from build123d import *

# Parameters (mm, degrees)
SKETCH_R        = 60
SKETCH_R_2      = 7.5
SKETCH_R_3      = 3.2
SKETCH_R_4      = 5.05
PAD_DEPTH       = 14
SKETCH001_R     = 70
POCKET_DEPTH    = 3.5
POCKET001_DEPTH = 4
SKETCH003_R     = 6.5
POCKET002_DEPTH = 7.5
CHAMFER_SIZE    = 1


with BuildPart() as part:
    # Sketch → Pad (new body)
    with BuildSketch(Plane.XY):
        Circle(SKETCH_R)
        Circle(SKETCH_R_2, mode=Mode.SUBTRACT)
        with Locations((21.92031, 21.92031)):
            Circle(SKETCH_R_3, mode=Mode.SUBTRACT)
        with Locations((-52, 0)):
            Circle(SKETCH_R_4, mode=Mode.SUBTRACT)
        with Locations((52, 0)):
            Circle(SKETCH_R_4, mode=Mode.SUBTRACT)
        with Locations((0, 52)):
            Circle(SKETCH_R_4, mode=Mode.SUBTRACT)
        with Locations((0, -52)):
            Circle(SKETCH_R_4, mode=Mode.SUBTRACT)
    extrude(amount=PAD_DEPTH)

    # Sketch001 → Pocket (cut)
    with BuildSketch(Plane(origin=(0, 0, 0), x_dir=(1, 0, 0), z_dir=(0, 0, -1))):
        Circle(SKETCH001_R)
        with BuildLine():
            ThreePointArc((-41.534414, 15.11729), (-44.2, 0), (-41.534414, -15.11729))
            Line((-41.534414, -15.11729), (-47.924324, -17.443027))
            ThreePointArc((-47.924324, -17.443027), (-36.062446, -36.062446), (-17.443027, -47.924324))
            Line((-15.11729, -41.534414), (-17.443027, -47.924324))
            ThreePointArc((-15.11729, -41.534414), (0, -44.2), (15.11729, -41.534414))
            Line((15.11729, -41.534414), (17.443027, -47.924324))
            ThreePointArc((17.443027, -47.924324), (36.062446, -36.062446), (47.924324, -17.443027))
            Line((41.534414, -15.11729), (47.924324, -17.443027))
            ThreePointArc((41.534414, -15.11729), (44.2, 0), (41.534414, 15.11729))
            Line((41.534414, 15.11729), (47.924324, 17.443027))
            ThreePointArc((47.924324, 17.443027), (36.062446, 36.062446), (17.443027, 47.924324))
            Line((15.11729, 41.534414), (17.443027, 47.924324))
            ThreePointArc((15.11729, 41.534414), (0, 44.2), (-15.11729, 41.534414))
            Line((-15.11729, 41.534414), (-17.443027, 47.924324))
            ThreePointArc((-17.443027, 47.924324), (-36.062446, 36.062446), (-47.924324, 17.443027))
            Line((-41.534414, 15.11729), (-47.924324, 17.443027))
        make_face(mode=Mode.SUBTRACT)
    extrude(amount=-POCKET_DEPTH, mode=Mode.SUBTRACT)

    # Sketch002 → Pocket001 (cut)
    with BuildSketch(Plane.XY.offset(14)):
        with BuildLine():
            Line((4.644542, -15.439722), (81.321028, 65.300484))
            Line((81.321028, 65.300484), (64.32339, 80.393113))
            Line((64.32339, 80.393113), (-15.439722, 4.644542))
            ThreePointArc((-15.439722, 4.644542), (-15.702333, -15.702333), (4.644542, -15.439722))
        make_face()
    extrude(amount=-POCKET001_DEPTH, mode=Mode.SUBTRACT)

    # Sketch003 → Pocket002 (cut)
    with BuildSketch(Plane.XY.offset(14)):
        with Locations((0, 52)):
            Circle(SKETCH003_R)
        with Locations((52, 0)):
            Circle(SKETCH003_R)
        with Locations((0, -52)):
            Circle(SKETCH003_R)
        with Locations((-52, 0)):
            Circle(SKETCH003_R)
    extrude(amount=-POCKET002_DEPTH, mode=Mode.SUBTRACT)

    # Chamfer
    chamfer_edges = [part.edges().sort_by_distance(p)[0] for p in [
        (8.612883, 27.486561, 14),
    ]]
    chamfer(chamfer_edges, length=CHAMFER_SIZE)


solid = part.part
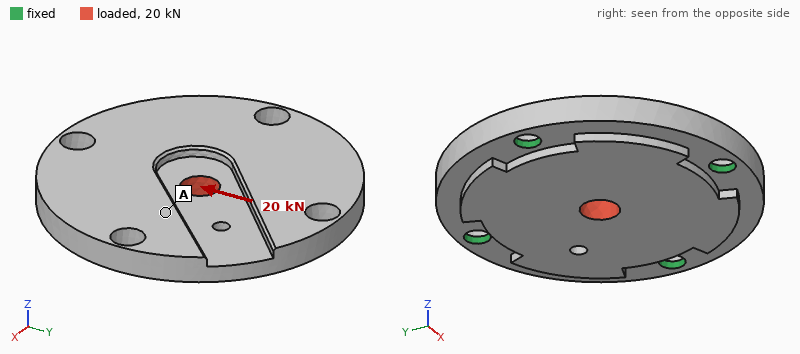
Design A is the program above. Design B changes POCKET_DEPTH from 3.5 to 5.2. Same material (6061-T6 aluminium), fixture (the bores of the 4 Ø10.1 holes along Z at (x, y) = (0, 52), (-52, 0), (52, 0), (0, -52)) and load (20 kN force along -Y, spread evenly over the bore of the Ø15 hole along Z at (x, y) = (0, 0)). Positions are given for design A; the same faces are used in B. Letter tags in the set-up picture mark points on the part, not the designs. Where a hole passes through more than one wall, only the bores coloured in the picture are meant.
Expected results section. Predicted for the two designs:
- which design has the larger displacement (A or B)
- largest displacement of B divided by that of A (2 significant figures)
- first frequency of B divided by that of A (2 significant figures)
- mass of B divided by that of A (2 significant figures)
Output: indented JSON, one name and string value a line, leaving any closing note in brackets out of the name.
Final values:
{
  "which design has the larger displacement": "B",
  "largest displacement of B divided by that of A": "1.3",
  "first frequency of B divided by that of A": "0.86",
  "mass of B divided by that of A": "0.95"
}
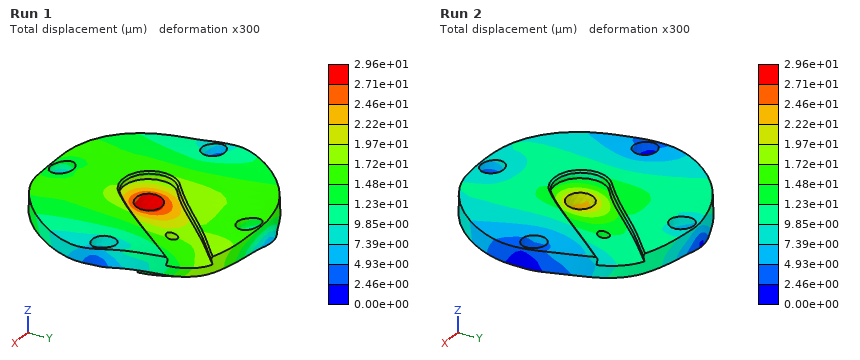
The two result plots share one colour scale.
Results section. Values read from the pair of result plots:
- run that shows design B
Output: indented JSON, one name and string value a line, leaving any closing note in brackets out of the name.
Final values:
{
  "run that shows design B": "Run 1"
}
